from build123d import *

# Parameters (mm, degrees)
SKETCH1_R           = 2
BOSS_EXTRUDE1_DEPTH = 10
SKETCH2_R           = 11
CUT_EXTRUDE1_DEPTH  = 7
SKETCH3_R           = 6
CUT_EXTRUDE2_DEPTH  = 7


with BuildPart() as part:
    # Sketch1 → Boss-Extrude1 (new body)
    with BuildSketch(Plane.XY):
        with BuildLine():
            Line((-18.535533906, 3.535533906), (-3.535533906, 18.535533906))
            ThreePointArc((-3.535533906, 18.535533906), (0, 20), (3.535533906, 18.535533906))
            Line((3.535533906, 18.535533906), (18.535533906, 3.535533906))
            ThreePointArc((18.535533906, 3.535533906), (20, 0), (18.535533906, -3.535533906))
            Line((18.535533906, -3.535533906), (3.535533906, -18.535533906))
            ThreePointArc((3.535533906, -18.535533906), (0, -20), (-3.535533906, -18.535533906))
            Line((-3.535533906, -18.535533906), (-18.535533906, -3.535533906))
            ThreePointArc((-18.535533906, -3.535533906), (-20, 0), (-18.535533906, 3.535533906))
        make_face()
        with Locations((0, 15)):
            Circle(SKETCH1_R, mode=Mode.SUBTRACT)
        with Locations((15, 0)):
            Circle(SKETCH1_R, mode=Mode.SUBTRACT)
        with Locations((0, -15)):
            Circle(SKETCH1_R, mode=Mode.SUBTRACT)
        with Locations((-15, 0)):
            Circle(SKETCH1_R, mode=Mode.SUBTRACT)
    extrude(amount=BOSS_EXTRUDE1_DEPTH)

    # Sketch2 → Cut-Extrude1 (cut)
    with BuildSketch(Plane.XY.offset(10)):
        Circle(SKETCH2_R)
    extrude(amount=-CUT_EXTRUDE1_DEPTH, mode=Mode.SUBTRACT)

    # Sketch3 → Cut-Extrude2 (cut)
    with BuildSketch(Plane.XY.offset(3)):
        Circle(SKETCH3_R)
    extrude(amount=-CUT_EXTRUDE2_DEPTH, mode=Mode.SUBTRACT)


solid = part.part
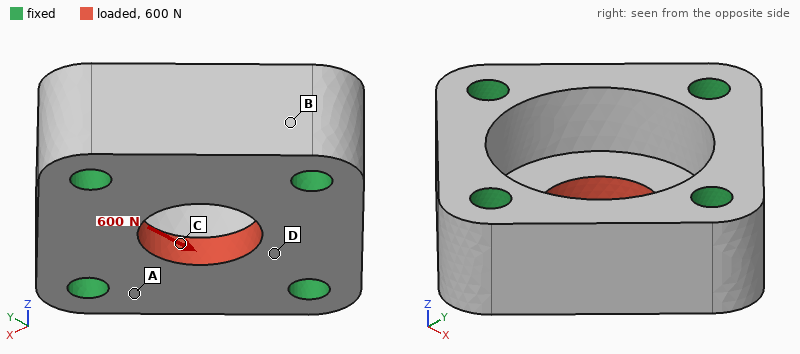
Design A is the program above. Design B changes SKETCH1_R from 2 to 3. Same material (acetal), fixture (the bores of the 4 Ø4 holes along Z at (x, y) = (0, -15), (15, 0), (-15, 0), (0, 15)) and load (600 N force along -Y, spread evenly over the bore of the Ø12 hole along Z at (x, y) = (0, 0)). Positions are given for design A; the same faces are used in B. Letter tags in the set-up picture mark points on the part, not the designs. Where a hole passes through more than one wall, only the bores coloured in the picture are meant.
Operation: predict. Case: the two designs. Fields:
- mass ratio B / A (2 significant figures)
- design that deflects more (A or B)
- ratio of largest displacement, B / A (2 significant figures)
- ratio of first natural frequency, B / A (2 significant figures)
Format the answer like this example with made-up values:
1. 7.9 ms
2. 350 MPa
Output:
1. 0.90
2. A
3. 0.87
4. 1.1
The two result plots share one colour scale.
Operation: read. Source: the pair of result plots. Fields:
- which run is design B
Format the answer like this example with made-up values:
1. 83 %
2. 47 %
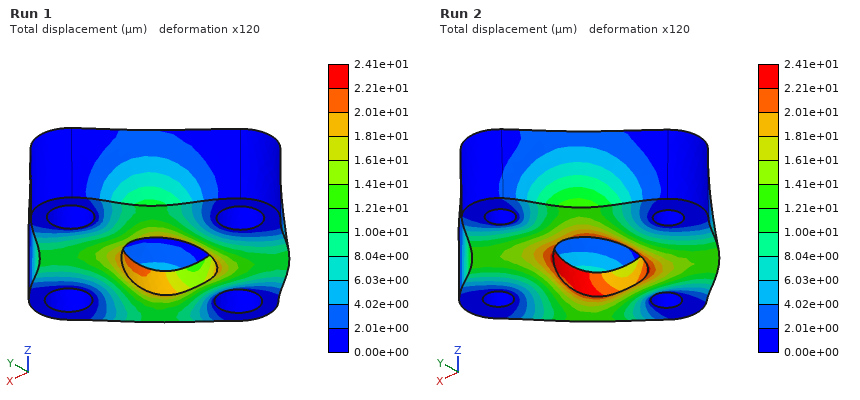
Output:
1. Run 1
